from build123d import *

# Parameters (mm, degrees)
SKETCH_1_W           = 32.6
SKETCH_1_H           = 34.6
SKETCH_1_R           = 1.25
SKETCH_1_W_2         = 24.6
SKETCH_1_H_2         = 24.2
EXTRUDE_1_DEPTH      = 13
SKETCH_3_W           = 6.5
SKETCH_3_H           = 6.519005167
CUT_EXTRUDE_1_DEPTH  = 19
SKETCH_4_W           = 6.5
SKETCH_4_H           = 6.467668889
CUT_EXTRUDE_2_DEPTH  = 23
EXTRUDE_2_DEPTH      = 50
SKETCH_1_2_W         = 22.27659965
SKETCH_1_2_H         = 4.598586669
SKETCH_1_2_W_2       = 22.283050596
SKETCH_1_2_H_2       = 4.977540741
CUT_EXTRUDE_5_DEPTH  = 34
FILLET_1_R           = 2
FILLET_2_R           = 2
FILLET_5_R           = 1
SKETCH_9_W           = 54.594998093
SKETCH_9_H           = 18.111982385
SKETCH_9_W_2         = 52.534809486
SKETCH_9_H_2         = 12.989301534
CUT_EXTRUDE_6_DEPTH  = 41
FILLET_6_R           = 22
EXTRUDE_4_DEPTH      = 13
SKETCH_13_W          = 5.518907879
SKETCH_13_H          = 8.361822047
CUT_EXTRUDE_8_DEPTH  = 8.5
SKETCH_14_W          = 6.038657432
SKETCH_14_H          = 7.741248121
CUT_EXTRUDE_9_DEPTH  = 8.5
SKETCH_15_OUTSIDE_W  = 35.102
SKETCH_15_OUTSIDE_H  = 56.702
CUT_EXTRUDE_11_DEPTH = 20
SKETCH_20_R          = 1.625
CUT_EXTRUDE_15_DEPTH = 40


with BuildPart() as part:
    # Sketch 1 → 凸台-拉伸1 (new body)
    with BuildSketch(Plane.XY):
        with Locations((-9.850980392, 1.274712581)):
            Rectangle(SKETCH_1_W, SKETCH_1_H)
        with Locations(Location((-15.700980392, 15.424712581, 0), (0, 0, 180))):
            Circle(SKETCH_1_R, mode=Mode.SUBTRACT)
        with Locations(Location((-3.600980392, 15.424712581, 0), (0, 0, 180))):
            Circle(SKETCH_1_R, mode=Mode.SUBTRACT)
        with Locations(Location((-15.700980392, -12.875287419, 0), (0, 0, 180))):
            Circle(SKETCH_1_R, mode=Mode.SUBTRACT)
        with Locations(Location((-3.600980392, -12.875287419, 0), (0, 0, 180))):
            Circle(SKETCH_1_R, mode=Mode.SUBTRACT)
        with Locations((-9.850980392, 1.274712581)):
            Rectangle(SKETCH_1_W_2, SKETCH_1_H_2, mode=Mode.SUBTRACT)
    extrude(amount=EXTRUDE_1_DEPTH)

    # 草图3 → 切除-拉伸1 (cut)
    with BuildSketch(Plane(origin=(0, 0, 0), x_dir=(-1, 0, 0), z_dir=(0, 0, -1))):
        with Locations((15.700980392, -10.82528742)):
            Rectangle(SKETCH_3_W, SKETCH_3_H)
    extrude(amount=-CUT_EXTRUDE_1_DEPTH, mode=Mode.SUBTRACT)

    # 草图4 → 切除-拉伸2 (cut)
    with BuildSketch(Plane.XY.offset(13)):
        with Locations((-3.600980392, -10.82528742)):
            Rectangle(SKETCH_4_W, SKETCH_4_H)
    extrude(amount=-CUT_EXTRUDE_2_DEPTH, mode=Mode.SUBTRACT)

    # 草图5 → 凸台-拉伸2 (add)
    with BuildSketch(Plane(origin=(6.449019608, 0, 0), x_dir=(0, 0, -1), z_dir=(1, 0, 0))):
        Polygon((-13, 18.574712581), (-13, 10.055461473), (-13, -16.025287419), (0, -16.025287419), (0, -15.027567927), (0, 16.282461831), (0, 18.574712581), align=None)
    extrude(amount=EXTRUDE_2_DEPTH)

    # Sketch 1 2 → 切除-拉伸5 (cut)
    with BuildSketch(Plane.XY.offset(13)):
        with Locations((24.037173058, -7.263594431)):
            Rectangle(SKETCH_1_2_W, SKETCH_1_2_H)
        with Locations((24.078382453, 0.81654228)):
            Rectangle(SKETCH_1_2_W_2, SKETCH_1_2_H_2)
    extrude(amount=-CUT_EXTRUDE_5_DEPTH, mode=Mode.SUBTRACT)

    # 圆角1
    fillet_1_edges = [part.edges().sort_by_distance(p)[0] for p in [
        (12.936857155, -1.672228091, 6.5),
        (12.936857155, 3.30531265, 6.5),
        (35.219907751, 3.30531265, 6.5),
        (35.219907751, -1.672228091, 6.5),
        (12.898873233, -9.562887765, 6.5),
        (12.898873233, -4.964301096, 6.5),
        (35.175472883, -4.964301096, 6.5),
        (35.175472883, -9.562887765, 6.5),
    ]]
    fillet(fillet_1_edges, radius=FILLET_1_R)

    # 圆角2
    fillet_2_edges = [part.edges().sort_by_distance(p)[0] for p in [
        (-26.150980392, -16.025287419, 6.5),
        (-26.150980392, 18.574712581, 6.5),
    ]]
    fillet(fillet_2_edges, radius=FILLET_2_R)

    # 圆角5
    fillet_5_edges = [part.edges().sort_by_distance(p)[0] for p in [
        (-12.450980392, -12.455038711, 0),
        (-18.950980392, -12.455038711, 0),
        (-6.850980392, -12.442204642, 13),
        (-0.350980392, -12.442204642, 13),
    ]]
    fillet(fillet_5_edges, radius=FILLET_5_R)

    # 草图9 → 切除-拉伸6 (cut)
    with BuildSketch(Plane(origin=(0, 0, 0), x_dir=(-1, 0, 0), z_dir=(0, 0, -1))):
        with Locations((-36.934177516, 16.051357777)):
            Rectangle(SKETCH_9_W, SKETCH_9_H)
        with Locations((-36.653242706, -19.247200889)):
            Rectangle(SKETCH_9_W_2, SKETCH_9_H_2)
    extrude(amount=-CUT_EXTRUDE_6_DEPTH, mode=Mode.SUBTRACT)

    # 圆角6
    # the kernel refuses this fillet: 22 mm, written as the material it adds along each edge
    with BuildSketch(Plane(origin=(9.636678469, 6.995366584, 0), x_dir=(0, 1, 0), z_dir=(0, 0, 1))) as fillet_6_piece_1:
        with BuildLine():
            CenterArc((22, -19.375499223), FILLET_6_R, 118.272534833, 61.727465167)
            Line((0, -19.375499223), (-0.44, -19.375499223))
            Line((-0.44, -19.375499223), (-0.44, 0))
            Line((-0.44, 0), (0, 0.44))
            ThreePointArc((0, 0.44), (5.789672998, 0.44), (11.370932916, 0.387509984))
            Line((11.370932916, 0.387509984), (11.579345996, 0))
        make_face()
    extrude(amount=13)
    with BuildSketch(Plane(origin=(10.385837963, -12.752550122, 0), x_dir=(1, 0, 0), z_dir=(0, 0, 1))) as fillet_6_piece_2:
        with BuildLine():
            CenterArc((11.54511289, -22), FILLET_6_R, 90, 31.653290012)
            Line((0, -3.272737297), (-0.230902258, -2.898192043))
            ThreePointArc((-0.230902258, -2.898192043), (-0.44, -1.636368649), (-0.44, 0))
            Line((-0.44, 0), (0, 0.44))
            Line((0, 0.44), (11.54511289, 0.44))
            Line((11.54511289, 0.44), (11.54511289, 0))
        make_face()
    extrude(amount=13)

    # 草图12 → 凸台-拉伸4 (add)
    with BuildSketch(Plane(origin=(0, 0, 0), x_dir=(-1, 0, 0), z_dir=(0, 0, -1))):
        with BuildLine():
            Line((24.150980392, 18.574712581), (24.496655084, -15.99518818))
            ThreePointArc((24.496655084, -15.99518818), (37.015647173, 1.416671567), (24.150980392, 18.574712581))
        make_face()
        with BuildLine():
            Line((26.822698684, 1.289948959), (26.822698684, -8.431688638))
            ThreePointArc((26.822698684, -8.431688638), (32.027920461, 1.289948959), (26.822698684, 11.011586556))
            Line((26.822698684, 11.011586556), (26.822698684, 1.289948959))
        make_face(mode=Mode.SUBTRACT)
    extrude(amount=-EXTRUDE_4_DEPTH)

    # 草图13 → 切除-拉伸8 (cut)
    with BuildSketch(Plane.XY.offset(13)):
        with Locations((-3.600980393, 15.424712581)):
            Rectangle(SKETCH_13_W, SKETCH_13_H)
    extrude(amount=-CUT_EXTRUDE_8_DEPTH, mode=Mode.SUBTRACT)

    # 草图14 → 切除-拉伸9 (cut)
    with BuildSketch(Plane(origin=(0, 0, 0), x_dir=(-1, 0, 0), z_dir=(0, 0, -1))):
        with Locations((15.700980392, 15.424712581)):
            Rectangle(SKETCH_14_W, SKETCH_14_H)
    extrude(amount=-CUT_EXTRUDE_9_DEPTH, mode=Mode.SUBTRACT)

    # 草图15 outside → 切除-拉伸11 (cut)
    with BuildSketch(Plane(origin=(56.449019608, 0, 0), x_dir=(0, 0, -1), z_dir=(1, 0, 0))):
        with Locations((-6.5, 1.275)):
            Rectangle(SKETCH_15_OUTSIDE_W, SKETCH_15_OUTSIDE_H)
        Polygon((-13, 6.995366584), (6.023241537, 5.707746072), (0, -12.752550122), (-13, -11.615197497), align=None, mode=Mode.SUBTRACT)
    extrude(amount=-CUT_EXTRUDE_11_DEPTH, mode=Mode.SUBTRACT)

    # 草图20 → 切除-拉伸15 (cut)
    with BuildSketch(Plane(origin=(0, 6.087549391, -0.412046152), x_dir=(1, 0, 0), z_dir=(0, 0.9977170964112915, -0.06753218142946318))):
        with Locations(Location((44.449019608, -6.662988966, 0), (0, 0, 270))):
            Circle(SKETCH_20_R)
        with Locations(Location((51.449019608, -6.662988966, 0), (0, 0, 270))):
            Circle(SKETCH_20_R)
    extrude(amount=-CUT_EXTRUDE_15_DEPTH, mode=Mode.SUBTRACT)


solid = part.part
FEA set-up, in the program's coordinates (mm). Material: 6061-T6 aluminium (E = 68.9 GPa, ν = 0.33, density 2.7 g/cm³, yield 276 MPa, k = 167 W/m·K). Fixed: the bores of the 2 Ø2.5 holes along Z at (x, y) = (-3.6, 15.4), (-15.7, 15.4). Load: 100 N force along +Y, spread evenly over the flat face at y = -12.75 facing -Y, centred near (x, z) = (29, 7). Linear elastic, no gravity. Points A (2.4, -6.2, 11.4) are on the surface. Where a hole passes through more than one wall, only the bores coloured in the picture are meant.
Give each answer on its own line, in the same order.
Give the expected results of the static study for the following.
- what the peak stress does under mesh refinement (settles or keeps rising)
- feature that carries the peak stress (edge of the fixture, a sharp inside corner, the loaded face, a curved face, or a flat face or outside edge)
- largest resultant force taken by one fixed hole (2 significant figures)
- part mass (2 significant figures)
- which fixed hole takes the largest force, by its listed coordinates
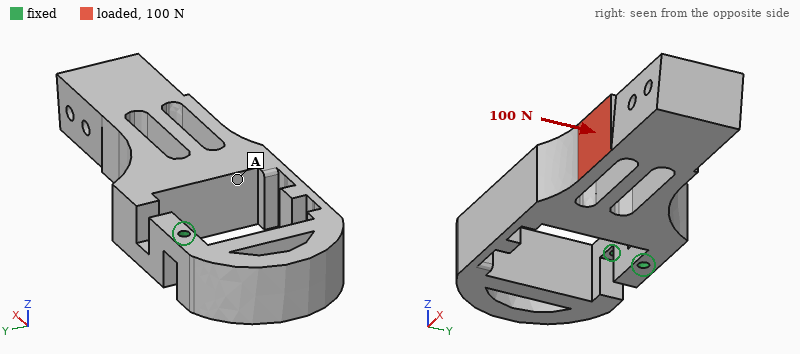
keeps rising
edge of the fixture
160 N
53 g
(-3.6, 15.4)
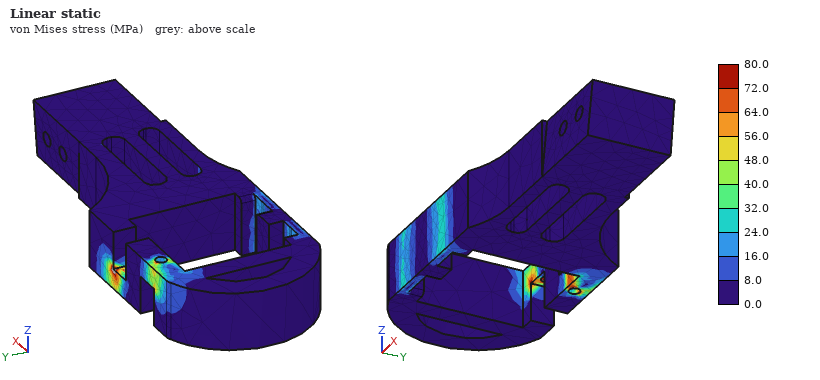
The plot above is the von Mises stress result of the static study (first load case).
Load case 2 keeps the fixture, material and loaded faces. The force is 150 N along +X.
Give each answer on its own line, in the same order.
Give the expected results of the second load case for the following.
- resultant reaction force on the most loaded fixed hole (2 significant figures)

120 N
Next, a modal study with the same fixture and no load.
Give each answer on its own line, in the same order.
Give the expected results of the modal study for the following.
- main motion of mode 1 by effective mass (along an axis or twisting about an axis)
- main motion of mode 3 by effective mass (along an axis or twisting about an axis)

along Z
along Z
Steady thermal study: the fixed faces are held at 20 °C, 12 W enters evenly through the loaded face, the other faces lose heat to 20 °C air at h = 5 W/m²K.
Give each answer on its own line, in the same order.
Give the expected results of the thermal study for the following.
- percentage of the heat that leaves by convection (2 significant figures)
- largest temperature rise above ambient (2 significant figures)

6.4 %
32 K
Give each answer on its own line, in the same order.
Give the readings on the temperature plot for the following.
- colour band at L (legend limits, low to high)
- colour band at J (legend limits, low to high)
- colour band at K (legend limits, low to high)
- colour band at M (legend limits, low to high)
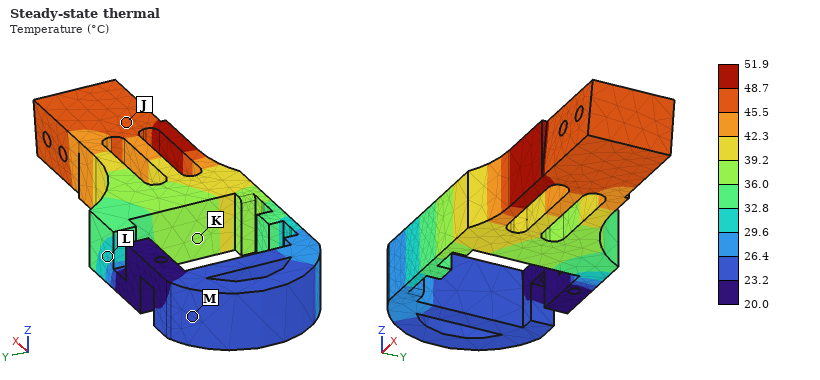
29.6 to 32.8 °C
45.5 to 48.7 °C
36.0 to 39.2 °C
23.2 to 26.4 °C
